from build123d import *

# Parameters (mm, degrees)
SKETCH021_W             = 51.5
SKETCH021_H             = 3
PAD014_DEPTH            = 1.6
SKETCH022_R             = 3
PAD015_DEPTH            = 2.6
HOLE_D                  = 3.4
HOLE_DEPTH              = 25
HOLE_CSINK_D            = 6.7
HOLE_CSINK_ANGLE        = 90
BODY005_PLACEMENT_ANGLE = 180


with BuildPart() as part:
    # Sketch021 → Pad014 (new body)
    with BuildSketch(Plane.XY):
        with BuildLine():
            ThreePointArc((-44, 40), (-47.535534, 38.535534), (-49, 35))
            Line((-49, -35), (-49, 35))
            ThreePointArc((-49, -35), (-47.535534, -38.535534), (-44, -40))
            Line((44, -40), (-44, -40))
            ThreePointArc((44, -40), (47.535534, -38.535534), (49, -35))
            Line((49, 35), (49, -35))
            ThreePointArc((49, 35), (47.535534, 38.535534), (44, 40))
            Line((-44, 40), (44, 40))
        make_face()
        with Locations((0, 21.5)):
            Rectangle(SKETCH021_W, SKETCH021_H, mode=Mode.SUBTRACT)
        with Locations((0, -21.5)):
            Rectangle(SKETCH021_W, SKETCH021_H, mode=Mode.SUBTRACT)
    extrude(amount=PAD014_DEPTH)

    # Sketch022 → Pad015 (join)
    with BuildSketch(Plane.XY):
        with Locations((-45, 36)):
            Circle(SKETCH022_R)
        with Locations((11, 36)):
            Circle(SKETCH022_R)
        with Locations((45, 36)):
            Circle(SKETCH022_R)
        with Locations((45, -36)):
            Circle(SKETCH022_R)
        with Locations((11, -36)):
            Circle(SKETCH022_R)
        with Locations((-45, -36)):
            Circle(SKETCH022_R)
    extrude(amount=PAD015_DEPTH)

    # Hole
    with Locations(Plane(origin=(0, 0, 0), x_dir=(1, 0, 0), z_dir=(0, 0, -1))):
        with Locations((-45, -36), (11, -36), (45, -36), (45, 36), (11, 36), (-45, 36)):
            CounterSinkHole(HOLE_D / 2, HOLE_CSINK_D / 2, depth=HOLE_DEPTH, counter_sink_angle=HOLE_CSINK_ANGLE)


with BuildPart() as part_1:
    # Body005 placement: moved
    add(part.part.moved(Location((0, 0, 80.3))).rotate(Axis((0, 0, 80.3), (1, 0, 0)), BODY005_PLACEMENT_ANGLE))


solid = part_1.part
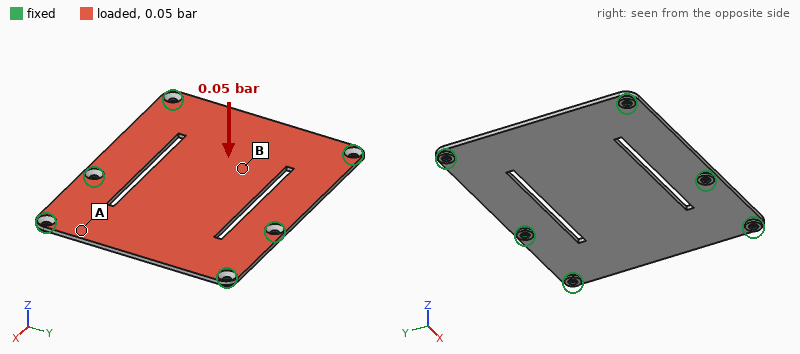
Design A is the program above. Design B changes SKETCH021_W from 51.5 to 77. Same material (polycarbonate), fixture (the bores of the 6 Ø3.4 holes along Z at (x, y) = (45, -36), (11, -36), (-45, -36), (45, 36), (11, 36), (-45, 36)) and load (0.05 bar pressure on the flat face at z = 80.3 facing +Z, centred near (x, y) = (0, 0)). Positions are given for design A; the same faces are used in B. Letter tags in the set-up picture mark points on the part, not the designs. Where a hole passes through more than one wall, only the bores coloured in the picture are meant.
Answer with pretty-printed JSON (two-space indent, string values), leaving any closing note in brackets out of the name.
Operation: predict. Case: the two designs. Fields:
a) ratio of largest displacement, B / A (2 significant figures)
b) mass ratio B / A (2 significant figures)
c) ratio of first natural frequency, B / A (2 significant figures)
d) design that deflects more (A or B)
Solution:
{
  "ratio of largest displacement, B / A": "2.0",
  "mass ratio B / A": "0.98",
  "ratio of first natural frequency, B / A": "0.69",
  "design that deflects more": "B"
}
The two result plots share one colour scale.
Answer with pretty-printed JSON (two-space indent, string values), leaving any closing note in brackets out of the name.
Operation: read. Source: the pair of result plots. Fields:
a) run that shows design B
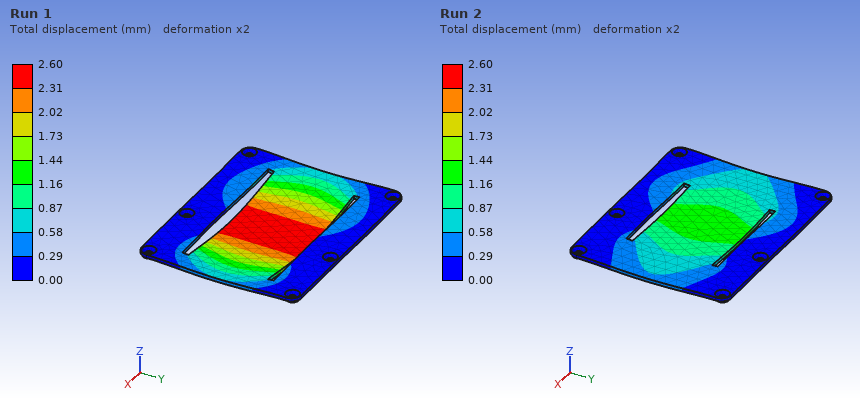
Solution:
{
  "run that shows design B": "Run 1"
}
